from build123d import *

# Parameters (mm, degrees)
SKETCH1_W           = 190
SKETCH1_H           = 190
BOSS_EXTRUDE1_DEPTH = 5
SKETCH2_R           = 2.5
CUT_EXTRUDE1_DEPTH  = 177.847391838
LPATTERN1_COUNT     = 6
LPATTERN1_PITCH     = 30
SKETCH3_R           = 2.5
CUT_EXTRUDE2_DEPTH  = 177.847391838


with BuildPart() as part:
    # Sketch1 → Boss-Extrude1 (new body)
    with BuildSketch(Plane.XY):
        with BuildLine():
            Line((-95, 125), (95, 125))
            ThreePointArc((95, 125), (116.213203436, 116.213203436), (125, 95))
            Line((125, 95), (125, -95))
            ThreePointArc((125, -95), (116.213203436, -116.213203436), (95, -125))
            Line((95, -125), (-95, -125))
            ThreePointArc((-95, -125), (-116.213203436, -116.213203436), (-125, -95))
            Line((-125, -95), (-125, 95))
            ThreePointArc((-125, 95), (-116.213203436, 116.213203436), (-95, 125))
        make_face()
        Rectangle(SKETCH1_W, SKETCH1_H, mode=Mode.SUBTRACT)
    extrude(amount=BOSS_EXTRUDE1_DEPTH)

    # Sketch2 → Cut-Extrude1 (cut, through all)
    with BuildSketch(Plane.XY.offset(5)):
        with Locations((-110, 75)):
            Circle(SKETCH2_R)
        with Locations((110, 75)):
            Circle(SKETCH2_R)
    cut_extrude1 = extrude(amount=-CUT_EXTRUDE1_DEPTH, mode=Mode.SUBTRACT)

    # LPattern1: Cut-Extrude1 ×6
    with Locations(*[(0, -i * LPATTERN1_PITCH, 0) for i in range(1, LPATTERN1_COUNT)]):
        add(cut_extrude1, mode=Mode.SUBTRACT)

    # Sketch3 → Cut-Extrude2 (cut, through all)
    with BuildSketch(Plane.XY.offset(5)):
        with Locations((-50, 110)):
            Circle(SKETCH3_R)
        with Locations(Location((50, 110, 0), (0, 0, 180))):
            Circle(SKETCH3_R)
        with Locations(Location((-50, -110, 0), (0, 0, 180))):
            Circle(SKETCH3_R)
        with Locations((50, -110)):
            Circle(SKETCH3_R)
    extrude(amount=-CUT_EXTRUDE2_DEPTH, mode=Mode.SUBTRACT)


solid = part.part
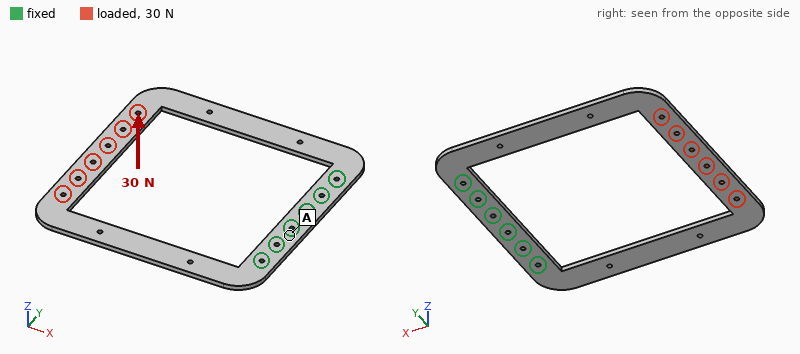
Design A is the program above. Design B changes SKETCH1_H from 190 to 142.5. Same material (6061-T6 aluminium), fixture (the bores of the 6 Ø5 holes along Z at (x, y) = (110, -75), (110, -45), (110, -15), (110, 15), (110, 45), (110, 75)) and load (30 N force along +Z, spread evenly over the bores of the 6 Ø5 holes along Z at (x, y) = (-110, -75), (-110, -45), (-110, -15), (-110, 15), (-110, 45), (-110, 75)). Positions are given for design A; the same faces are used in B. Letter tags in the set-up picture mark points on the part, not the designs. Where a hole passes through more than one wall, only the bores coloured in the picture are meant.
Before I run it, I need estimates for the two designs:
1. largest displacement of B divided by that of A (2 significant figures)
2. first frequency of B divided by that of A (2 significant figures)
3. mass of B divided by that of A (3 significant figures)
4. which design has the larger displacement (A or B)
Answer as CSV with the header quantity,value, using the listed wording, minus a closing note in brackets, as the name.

quantity,value
largest displacement of B divided by that of A,0.53
first frequency of B divided by that of A,1.3
mass of B divided by that of A,1.36
which design has the larger displacement,A
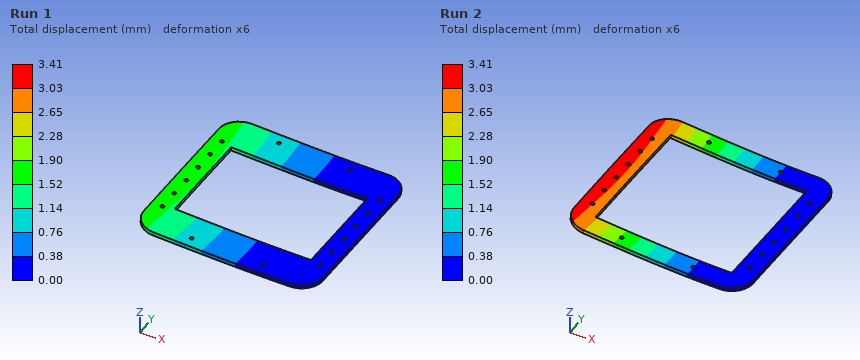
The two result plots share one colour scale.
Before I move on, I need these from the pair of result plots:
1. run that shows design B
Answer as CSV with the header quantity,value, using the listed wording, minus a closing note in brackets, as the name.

quantity,value
run that shows design B,Run 1
